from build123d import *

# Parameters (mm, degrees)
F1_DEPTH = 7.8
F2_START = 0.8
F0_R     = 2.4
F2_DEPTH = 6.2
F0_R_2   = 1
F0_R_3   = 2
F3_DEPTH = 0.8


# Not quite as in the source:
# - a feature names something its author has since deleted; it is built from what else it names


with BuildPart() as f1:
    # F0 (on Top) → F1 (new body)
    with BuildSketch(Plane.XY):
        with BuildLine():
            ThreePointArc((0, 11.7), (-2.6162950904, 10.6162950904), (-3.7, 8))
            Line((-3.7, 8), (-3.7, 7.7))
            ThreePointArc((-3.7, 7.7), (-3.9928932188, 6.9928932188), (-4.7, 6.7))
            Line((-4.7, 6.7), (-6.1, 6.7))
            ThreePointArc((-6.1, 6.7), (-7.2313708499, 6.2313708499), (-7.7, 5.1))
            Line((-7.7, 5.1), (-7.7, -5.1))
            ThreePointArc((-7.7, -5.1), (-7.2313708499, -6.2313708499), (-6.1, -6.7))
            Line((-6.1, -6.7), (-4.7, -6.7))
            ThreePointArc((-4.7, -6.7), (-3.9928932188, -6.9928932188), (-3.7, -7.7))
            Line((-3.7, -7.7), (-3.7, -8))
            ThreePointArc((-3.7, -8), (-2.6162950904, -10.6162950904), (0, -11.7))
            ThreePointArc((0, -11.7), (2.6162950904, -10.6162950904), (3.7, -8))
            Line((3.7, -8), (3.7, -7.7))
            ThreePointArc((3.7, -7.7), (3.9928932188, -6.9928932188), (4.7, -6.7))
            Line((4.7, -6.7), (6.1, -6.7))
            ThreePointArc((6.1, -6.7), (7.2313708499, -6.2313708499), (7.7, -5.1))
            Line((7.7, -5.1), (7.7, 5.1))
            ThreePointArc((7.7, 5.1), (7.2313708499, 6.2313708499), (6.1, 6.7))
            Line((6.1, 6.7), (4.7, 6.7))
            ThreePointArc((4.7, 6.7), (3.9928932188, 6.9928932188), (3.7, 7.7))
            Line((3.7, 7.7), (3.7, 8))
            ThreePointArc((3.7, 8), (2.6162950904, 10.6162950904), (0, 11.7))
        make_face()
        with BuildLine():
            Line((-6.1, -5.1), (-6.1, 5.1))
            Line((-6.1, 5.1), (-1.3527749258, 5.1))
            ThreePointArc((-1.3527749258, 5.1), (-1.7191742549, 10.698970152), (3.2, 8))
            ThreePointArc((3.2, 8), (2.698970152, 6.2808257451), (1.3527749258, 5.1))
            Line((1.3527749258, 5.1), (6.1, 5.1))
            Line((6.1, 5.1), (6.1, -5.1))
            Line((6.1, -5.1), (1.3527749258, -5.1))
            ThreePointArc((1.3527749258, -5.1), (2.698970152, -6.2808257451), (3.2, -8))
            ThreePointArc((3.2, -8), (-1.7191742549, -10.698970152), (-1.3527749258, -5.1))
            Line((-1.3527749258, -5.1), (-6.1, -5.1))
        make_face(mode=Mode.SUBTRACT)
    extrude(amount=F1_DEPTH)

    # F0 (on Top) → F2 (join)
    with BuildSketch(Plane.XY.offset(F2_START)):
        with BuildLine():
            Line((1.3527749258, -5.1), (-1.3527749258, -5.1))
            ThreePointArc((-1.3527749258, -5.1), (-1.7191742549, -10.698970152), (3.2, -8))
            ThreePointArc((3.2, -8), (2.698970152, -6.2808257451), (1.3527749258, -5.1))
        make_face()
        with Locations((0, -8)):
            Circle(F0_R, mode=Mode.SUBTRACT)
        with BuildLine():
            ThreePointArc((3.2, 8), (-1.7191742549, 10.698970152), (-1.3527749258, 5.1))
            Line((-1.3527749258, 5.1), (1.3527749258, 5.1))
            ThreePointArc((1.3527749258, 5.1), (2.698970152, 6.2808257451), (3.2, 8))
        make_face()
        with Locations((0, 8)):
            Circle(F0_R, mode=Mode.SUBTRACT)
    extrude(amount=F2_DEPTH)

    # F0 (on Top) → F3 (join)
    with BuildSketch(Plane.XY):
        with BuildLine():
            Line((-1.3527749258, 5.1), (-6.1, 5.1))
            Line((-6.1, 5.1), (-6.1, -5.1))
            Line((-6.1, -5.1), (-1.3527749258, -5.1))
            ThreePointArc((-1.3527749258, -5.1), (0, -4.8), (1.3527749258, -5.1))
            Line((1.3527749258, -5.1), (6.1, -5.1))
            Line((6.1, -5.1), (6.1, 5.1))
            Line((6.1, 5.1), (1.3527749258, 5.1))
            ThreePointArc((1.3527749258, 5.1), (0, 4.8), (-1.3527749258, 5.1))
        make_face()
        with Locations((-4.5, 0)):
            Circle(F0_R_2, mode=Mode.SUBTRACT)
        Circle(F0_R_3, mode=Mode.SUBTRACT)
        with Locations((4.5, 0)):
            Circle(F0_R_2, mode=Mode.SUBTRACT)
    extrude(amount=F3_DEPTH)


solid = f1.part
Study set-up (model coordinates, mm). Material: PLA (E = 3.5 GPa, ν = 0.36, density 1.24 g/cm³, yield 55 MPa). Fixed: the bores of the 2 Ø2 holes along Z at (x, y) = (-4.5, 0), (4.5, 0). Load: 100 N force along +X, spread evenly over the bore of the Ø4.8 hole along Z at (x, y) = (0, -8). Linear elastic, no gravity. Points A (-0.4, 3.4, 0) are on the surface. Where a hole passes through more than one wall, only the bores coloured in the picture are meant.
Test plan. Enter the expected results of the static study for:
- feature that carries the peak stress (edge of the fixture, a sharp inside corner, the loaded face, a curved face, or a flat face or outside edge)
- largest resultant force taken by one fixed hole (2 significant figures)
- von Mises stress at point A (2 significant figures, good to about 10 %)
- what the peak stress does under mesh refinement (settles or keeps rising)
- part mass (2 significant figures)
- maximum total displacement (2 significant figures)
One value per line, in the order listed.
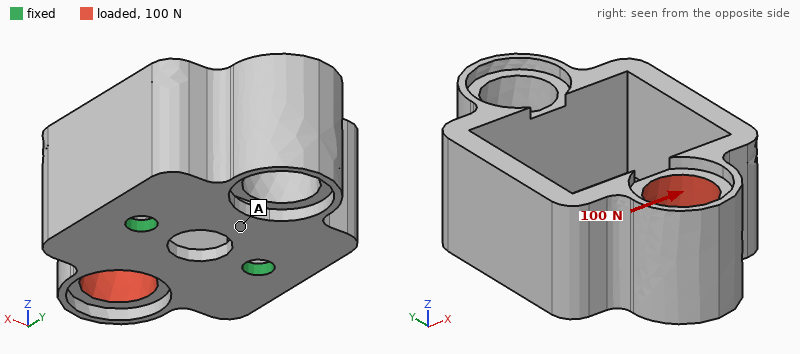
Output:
edge of the fixture
89 N
8.8 MPa
keeps rising
1.1 g
0.19 mm
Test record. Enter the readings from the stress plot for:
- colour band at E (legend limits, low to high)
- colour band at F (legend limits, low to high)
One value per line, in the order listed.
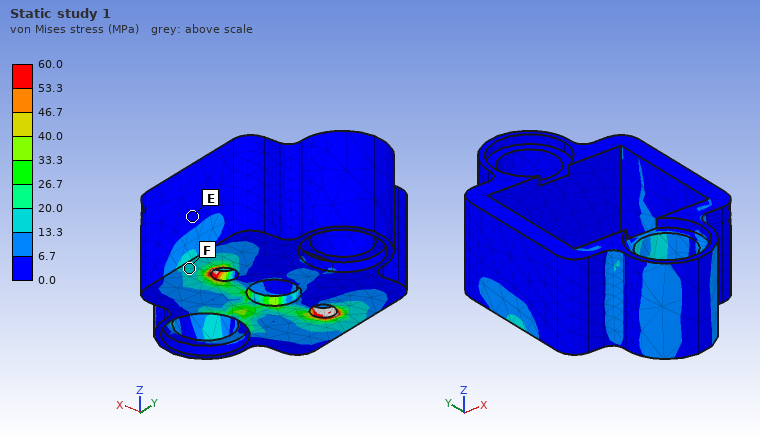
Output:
0.0 to 6.7 MPa
13.3 to 20.0 MPa
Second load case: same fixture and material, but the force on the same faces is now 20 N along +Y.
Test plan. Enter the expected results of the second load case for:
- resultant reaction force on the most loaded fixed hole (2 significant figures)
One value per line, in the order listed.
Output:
10 N
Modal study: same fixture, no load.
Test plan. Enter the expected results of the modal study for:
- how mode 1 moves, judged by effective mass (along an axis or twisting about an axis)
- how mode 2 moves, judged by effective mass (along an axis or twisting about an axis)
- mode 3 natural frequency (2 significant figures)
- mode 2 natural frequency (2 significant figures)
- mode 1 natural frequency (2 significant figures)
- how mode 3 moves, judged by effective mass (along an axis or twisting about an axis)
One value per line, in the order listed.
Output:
along Y
along X
6800 Hz
5500 Hz
1600 Hz
along Z
